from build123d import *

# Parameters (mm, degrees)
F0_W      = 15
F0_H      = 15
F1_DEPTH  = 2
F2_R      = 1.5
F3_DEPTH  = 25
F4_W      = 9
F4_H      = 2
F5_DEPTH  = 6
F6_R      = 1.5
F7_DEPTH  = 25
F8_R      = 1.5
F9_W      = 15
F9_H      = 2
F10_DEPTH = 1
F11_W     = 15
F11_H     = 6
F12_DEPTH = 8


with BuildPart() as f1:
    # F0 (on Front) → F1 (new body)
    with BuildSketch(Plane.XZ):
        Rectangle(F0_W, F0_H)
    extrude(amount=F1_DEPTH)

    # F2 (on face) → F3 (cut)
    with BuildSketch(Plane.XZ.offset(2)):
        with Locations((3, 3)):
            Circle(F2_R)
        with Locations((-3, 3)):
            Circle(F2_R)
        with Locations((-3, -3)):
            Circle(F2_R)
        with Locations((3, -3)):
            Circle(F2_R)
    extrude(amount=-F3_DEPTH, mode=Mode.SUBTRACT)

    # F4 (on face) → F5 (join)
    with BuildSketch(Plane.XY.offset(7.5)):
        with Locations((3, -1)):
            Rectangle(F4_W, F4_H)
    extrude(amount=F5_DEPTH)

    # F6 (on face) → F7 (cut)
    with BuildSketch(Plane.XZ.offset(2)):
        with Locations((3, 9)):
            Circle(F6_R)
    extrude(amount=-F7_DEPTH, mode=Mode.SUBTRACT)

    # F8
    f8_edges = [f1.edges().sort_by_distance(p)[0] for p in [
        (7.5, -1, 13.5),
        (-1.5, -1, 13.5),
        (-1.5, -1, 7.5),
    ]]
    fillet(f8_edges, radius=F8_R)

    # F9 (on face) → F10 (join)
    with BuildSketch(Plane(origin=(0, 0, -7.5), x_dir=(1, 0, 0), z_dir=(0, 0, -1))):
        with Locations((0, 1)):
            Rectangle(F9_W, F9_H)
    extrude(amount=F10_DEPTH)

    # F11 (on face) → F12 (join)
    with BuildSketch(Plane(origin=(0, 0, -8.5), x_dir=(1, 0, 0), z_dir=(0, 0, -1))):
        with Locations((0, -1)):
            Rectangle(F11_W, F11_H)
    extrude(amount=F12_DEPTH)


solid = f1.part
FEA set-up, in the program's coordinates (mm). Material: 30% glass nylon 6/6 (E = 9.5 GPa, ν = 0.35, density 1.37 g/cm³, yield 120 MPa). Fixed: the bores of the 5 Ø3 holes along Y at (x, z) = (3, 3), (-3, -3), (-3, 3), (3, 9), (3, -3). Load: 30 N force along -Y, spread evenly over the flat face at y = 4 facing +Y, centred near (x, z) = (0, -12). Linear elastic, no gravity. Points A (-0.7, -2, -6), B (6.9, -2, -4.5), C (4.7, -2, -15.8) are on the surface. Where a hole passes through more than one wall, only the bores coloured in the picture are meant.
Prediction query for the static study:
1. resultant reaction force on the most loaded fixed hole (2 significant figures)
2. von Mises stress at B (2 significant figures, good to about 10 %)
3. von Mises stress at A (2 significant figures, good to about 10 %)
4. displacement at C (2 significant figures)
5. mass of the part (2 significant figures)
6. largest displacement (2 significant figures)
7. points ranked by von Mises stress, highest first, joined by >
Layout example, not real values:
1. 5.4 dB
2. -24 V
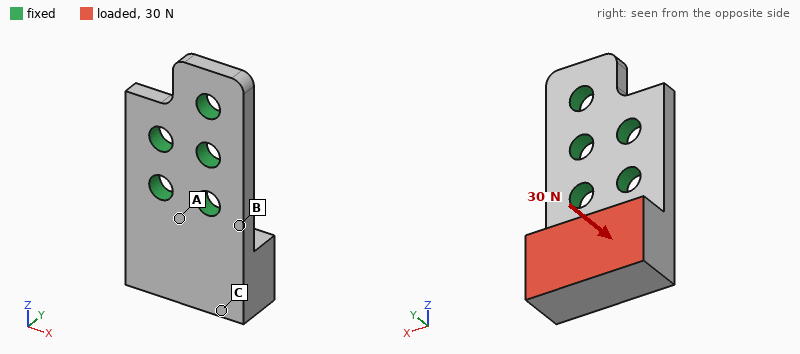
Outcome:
1. 17 N
2. 13 MPa
3. 17 MPa
4. 0.095 mm
5. 1.7 g
6. 0.11 mm
7. A > B > C
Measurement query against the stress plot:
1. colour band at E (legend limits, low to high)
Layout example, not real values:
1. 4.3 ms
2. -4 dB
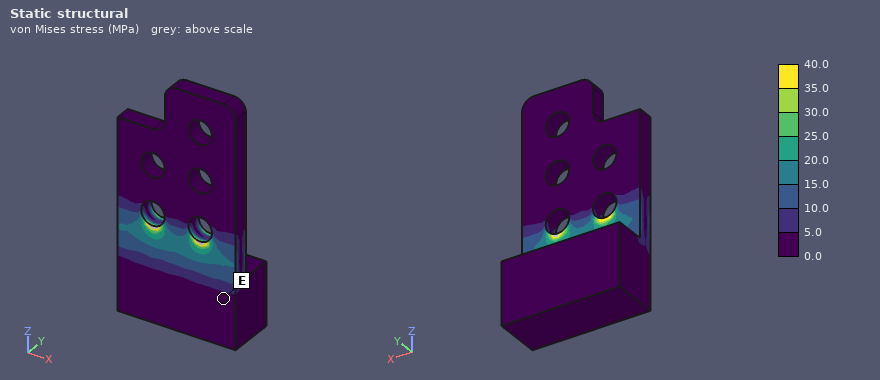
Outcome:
1. 0.0 to 5.0 MPa
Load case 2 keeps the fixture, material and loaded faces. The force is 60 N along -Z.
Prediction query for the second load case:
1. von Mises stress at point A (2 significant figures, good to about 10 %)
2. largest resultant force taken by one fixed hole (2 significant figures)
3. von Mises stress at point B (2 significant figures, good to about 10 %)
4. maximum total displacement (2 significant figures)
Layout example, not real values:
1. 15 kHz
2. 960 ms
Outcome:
1. 24 MPa
2. 28 N
3. 17 MPa
4. 0.18 mm
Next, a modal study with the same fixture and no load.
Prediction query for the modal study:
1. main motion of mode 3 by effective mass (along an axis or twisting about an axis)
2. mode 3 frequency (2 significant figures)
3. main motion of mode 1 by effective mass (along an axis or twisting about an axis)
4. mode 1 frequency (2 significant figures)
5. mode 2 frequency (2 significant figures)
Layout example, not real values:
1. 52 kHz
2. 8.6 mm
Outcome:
1. along X
2. 13 kHz
3. along Y
4. 3100 Hz
5. 8400 Hz
